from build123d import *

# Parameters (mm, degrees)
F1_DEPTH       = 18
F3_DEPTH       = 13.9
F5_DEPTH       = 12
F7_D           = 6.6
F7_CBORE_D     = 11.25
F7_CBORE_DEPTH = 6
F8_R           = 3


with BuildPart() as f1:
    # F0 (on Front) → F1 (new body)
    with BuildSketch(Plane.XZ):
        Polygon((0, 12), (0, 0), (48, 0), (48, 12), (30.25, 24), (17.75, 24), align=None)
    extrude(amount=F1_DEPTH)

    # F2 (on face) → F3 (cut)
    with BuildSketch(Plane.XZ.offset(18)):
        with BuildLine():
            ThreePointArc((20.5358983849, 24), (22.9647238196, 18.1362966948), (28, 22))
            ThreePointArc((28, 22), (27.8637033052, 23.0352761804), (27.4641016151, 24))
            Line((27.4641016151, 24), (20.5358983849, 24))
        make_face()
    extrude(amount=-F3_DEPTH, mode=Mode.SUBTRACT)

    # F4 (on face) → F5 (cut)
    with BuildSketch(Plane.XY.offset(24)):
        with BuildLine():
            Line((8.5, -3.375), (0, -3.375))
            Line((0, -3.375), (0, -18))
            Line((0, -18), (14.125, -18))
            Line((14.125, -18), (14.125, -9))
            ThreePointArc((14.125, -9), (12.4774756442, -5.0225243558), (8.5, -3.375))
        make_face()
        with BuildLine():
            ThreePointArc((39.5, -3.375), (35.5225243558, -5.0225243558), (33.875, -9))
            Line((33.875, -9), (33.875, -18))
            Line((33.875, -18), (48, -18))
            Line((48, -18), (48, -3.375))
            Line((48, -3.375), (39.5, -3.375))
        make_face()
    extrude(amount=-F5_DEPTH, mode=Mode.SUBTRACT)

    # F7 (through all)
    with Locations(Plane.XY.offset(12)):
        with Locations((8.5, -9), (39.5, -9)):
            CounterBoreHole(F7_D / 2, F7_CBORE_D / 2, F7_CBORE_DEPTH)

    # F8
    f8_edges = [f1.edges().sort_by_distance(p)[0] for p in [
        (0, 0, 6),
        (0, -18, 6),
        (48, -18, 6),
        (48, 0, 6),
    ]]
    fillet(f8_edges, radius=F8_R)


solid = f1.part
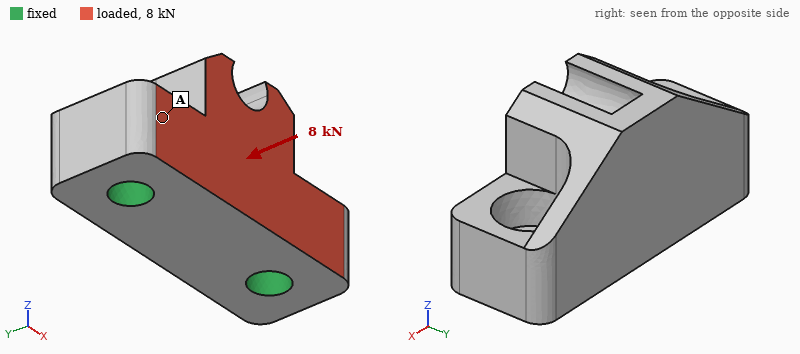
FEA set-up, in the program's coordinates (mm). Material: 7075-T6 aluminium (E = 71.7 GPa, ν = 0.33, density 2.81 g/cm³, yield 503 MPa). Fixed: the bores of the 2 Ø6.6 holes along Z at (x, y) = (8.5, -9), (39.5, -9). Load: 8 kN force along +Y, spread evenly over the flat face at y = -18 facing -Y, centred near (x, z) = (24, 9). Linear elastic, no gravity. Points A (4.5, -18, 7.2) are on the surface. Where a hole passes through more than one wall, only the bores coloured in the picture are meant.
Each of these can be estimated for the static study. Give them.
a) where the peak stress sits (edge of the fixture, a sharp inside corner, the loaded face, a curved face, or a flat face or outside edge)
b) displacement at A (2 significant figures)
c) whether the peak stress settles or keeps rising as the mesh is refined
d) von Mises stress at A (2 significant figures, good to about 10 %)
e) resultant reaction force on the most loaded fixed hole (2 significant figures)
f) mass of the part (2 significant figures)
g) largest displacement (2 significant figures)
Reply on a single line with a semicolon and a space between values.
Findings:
edge of the fixture; 13 µm; keeps rising; 33 MPa; 4.0 kN; 36 g; 57 µm
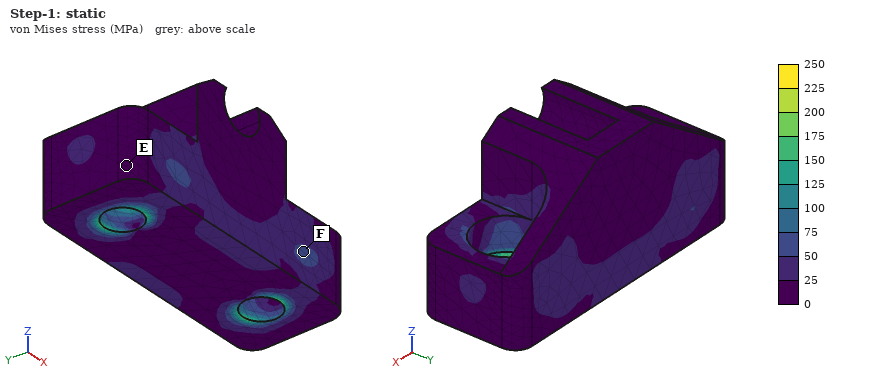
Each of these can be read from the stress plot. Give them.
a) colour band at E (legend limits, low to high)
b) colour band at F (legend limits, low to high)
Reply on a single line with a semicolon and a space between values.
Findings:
0 to 25 MPa; 50 to 75 MPa
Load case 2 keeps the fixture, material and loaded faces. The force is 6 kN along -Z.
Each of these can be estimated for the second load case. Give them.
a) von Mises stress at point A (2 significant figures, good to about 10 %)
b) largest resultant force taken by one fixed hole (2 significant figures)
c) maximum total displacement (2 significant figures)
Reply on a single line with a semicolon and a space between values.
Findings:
29 MPa; 3.1 kN; 54 µm
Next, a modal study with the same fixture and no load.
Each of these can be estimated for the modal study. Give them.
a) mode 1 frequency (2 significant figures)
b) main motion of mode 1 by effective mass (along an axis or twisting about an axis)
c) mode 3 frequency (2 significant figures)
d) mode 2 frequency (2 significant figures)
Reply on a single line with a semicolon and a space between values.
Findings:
12 kHz; along Y; 27 kHz; 27 kHz
